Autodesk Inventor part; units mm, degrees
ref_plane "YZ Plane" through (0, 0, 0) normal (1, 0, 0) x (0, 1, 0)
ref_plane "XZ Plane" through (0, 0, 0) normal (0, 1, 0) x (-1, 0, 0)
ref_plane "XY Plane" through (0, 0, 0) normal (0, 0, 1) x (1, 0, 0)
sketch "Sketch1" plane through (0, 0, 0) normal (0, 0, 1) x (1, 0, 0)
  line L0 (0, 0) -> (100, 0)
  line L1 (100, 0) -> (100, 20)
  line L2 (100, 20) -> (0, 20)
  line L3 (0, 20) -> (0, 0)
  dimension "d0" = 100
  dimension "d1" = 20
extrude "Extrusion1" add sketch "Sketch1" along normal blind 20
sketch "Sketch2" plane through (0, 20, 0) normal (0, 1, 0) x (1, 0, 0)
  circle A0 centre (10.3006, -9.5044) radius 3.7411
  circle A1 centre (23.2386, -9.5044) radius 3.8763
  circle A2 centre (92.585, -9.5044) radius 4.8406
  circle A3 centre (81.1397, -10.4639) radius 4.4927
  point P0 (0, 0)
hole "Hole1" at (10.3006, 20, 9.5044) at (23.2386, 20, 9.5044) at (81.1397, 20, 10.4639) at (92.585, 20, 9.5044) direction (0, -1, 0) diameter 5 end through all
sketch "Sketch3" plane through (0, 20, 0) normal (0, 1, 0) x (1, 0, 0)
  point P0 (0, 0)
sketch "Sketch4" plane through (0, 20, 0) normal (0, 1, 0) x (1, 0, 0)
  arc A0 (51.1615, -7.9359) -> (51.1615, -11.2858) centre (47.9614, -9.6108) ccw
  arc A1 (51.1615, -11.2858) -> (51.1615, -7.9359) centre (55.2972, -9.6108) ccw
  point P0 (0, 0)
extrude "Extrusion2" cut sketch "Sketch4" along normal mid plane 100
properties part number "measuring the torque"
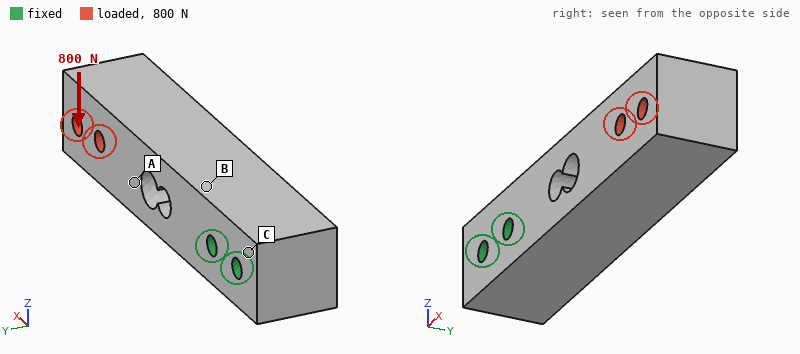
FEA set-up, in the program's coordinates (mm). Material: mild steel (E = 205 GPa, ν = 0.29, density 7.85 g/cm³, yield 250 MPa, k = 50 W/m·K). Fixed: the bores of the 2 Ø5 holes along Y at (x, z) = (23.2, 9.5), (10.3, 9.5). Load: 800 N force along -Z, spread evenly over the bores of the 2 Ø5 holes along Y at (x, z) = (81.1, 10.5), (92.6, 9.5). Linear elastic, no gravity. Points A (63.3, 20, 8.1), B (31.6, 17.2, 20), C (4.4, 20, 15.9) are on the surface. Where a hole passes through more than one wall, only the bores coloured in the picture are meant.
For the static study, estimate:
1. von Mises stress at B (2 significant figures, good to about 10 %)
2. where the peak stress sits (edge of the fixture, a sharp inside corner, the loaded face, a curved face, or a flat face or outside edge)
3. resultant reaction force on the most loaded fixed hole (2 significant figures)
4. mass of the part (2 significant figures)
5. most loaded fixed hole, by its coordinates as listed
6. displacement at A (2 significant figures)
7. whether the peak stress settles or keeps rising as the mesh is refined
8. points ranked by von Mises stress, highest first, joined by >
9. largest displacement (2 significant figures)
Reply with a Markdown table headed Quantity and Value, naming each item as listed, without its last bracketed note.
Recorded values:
| Quantity | Value |
|---|---|
| von Mises stress at B | 34 MPa |
| where the peak stress sits | edge of the fixture |
| resultant reaction force on the most loaded fixed hole | 3.0 kN |
| mass of the part | 290 g |
| most loaded fixed hole, by its coordinates as listed | (23.2, 9.5) |
| displacement at A | 21 µm |
| whether the peak stress settles or keeps rising as the mesh is refined | keeps rising |
| points ranked by von Mises stress, highest first, joined by > | B > A > C |
| largest displacement | 49 µm |
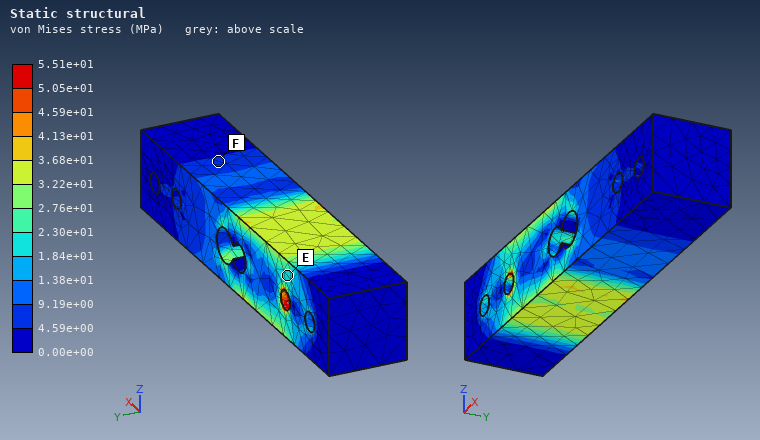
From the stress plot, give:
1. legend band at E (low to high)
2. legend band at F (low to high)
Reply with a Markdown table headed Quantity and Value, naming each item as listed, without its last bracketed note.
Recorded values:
| Quantity | Value |
|---|---|
| legend band at E | 1.84e+01 to 2.30e+01 MPa |
| legend band at F | 4.59e+00 to 9.19e+00 MPa |
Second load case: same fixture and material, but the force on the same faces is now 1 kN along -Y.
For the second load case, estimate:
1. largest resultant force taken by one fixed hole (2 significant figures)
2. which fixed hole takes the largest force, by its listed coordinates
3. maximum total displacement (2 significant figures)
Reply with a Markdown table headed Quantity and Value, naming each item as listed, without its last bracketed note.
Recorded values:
| Quantity | Value |
|---|---|
| largest resultant force taken by one fixed hole | 1.6 kN |
| which fixed hole takes the largest force, by its listed coordinates | (23.2, 9.5) |
| maximum total displacement | 55 µm |
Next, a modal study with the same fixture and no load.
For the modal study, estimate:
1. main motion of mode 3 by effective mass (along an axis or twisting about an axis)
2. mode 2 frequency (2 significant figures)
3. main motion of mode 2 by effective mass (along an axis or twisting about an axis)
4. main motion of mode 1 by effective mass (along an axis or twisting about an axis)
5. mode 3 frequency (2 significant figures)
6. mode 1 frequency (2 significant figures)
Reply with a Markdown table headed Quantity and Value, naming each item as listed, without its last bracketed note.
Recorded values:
| Quantity | Value |
|---|---|
| main motion of mode 3 by effective mass | twisting about X |
| mode 2 frequency | 2500 Hz |
| main motion of mode 2 by effective mass | along Y |
| main motion of mode 1 by effective mass | along Z |
| mode 3 frequency | 8300 Hz |
| mode 1 frequency | 2300 Hz |
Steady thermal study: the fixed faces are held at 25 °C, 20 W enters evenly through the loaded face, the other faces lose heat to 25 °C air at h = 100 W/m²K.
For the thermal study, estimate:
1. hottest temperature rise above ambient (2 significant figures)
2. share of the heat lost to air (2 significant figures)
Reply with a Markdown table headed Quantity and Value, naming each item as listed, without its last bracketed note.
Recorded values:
| Quantity | Value |
|---|---|
| hottest temperature rise above ambient | 36 K |
| share of the heat lost to air | 66 % |
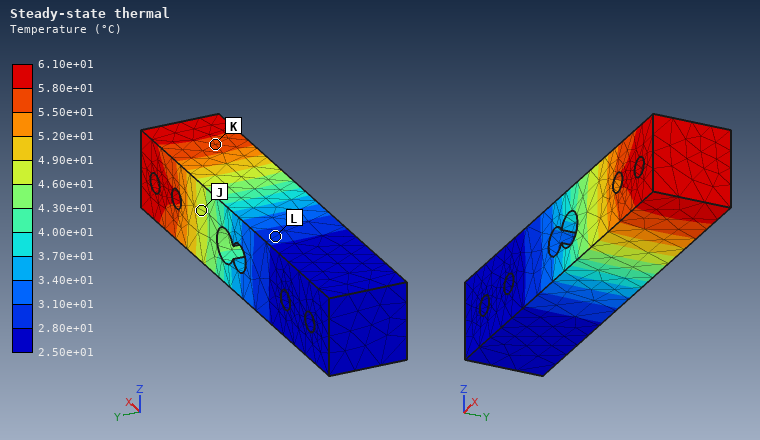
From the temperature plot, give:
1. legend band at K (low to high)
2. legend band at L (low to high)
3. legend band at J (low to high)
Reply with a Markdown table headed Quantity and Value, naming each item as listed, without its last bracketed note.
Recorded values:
| Quantity | Value |
|---|---|
| legend band at K | 5.50e+01 to 5.80e+01 °C |
| legend band at L | 2.80e+01 to 3.10e+01 °C |
| legend band at J | 4.60e+01 to 4.90e+01 °C |
